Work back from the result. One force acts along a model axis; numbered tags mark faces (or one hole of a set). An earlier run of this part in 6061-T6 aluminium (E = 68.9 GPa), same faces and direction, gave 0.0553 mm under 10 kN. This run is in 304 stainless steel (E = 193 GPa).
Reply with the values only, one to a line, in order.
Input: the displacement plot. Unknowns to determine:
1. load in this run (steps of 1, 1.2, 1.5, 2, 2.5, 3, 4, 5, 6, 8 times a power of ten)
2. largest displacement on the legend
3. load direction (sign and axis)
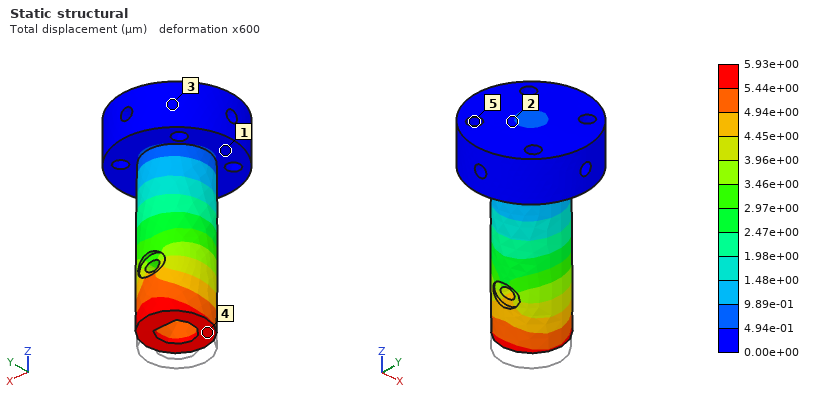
3 kN
5.93e+00 µm
+Z
